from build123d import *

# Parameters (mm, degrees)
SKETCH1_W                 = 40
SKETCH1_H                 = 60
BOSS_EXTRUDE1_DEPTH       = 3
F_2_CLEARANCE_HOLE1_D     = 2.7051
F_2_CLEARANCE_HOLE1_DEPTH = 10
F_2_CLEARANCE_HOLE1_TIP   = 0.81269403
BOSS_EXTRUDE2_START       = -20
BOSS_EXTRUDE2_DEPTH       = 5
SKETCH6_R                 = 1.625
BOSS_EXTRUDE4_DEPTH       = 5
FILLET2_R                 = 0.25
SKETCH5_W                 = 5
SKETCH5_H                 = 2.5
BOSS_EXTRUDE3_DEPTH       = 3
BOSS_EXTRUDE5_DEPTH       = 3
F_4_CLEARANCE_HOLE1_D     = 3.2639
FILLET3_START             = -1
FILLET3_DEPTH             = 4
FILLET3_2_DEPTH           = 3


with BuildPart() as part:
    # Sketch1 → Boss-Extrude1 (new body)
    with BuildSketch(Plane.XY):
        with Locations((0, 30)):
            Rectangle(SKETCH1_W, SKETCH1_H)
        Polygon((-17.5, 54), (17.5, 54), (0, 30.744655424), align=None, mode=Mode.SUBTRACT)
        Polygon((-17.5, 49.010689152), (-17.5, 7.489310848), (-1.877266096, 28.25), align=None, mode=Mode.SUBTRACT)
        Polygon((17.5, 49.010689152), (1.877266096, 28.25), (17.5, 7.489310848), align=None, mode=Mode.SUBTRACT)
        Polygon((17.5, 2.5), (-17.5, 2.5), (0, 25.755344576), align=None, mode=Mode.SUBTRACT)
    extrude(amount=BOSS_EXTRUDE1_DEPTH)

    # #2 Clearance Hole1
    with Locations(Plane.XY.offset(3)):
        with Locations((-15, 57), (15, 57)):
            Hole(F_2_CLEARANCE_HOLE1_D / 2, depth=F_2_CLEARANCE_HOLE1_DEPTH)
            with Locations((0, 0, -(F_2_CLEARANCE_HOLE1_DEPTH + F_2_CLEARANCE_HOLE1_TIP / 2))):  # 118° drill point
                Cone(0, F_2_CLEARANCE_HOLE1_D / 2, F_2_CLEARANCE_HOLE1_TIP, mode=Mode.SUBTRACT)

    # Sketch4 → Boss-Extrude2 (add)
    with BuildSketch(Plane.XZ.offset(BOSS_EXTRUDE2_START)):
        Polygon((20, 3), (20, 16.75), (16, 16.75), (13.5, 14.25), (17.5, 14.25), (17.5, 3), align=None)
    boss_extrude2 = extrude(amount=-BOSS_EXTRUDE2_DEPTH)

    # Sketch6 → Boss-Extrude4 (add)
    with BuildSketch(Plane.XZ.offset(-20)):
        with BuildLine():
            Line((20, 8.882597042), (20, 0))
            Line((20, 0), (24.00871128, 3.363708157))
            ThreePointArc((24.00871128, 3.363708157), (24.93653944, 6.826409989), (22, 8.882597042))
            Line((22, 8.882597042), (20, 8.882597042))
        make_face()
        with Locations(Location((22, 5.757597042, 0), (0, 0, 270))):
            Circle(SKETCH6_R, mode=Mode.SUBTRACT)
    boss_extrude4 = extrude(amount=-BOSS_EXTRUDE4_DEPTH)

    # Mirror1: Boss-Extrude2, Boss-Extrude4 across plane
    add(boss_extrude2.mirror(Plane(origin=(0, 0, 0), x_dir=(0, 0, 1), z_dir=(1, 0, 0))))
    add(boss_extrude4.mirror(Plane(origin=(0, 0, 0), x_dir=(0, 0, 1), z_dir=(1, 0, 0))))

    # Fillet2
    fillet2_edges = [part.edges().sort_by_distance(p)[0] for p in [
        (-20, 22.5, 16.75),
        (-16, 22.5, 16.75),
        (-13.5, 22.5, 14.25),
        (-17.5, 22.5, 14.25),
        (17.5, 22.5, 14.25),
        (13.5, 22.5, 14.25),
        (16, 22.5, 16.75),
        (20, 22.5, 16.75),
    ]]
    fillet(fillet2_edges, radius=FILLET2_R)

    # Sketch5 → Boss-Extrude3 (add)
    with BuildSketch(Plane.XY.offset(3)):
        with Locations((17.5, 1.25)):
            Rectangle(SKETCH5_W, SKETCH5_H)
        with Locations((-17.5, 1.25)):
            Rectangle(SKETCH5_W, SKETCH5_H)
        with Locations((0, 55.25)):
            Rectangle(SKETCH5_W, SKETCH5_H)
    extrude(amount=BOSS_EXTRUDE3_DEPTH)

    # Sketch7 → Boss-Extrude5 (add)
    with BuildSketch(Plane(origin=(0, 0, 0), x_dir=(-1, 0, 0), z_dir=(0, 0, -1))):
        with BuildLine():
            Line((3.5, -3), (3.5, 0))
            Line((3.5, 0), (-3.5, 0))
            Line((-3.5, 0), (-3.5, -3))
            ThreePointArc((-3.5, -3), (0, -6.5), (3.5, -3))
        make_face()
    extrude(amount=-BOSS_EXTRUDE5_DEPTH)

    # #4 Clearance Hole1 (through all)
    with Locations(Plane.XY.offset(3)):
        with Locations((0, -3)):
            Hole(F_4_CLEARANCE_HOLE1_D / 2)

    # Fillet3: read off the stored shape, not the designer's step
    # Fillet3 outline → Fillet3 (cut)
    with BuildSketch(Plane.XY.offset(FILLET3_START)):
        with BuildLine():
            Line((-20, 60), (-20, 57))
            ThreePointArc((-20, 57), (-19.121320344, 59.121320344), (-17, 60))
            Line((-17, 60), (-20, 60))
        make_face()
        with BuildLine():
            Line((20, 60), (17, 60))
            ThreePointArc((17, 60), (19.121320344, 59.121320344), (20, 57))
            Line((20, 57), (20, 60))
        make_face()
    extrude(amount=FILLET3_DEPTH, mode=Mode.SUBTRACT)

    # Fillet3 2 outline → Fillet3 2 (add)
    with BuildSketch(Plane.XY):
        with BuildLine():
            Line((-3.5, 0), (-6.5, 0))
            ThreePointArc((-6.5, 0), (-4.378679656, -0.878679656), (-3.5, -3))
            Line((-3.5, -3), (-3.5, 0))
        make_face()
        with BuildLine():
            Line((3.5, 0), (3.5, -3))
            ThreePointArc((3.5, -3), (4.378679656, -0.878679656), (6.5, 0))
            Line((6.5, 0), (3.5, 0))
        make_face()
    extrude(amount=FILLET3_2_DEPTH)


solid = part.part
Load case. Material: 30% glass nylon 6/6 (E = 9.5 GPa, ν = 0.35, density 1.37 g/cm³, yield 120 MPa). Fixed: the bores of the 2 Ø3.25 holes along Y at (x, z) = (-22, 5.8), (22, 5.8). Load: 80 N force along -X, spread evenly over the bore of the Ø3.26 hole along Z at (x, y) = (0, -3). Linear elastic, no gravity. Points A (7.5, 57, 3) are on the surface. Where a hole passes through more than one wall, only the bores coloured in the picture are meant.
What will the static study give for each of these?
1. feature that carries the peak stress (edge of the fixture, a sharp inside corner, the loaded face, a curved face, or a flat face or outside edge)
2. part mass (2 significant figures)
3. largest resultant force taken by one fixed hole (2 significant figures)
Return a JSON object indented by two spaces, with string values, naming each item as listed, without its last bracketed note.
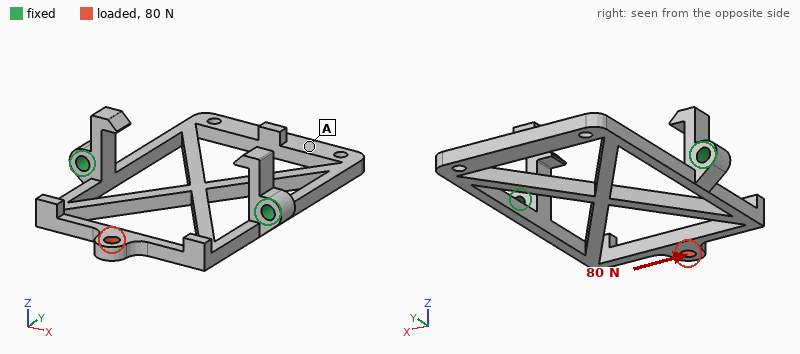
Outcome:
{
  "feature that carries the peak stress": "a flat face or outside edge",
  "part mass": "5.0 g",
  "largest resultant force taken by one fixed hole": "60 N"
}
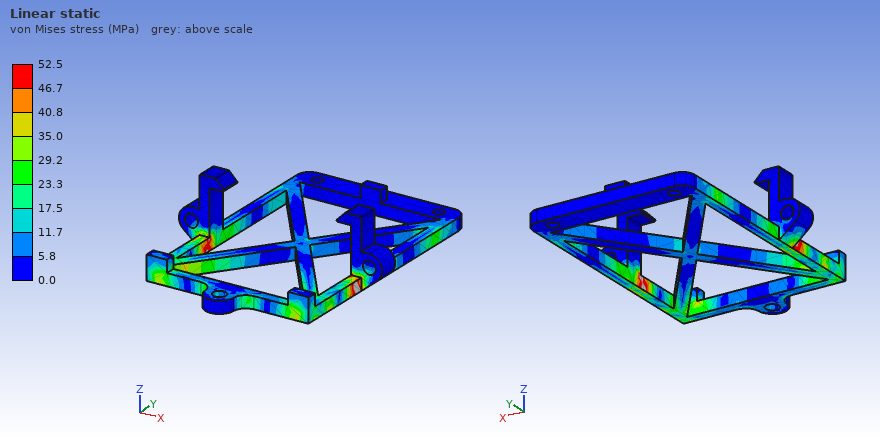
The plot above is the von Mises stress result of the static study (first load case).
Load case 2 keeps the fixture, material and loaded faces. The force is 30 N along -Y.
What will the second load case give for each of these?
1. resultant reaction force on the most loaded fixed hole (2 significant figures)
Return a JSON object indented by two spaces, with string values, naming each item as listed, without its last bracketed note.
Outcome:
{
  "resultant reaction force on the most loaded fixed hole": "16 N"
}
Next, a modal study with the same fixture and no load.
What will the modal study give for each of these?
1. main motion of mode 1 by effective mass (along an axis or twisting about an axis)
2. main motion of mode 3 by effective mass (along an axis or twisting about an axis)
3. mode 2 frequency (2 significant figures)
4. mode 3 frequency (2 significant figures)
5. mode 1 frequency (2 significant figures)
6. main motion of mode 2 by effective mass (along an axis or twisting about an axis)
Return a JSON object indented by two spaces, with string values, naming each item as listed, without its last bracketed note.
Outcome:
{
  "main motion of mode 1 by effective mass": "along Z",
  "main motion of mode 3 by effective mass": "along X",
  "mode 2 frequency": "1100 Hz",
  "mode 3 frequency": "1200 Hz",
  "mode 1 frequency": "470 Hz",
  "main motion of mode 2 by effective mass": "along Z"
}
